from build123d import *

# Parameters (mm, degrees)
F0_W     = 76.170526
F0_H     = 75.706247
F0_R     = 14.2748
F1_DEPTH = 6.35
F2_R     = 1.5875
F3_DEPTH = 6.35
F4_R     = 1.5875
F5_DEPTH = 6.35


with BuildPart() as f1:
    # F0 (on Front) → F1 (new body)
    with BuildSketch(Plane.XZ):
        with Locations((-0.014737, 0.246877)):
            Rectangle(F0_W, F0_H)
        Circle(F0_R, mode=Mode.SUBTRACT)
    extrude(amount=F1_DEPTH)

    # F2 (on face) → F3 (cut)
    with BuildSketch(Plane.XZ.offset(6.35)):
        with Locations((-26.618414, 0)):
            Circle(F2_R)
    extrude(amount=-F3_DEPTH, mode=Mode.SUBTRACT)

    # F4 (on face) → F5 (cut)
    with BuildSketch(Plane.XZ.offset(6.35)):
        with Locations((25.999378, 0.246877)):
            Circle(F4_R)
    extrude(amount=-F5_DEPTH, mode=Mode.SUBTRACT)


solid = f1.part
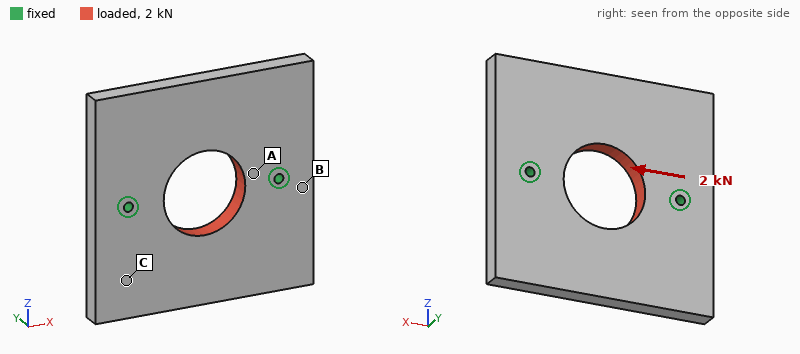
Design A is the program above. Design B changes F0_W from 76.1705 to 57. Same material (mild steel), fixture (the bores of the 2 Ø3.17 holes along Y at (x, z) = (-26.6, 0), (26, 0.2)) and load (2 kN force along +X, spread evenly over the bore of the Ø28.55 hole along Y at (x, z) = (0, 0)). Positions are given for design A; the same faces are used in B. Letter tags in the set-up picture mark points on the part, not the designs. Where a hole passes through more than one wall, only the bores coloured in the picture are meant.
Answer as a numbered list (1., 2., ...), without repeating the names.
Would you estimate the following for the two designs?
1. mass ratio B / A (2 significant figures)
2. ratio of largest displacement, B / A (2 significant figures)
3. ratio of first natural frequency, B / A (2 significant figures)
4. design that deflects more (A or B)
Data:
1. 0.72
2. 1.4
3. 0.93
4. B
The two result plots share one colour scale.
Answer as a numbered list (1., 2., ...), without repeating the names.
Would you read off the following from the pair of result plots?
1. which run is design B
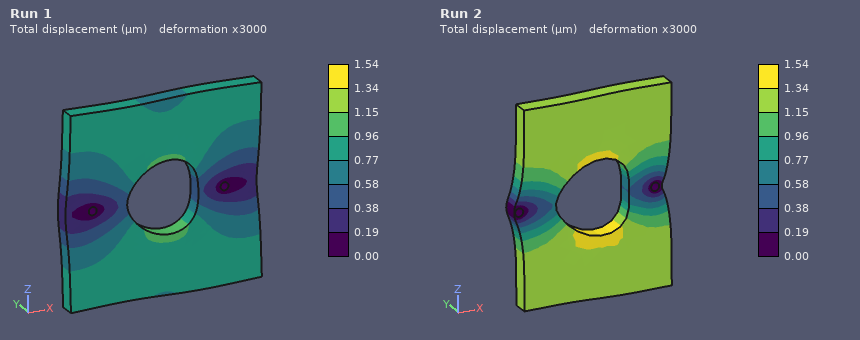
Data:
1. Run 2
